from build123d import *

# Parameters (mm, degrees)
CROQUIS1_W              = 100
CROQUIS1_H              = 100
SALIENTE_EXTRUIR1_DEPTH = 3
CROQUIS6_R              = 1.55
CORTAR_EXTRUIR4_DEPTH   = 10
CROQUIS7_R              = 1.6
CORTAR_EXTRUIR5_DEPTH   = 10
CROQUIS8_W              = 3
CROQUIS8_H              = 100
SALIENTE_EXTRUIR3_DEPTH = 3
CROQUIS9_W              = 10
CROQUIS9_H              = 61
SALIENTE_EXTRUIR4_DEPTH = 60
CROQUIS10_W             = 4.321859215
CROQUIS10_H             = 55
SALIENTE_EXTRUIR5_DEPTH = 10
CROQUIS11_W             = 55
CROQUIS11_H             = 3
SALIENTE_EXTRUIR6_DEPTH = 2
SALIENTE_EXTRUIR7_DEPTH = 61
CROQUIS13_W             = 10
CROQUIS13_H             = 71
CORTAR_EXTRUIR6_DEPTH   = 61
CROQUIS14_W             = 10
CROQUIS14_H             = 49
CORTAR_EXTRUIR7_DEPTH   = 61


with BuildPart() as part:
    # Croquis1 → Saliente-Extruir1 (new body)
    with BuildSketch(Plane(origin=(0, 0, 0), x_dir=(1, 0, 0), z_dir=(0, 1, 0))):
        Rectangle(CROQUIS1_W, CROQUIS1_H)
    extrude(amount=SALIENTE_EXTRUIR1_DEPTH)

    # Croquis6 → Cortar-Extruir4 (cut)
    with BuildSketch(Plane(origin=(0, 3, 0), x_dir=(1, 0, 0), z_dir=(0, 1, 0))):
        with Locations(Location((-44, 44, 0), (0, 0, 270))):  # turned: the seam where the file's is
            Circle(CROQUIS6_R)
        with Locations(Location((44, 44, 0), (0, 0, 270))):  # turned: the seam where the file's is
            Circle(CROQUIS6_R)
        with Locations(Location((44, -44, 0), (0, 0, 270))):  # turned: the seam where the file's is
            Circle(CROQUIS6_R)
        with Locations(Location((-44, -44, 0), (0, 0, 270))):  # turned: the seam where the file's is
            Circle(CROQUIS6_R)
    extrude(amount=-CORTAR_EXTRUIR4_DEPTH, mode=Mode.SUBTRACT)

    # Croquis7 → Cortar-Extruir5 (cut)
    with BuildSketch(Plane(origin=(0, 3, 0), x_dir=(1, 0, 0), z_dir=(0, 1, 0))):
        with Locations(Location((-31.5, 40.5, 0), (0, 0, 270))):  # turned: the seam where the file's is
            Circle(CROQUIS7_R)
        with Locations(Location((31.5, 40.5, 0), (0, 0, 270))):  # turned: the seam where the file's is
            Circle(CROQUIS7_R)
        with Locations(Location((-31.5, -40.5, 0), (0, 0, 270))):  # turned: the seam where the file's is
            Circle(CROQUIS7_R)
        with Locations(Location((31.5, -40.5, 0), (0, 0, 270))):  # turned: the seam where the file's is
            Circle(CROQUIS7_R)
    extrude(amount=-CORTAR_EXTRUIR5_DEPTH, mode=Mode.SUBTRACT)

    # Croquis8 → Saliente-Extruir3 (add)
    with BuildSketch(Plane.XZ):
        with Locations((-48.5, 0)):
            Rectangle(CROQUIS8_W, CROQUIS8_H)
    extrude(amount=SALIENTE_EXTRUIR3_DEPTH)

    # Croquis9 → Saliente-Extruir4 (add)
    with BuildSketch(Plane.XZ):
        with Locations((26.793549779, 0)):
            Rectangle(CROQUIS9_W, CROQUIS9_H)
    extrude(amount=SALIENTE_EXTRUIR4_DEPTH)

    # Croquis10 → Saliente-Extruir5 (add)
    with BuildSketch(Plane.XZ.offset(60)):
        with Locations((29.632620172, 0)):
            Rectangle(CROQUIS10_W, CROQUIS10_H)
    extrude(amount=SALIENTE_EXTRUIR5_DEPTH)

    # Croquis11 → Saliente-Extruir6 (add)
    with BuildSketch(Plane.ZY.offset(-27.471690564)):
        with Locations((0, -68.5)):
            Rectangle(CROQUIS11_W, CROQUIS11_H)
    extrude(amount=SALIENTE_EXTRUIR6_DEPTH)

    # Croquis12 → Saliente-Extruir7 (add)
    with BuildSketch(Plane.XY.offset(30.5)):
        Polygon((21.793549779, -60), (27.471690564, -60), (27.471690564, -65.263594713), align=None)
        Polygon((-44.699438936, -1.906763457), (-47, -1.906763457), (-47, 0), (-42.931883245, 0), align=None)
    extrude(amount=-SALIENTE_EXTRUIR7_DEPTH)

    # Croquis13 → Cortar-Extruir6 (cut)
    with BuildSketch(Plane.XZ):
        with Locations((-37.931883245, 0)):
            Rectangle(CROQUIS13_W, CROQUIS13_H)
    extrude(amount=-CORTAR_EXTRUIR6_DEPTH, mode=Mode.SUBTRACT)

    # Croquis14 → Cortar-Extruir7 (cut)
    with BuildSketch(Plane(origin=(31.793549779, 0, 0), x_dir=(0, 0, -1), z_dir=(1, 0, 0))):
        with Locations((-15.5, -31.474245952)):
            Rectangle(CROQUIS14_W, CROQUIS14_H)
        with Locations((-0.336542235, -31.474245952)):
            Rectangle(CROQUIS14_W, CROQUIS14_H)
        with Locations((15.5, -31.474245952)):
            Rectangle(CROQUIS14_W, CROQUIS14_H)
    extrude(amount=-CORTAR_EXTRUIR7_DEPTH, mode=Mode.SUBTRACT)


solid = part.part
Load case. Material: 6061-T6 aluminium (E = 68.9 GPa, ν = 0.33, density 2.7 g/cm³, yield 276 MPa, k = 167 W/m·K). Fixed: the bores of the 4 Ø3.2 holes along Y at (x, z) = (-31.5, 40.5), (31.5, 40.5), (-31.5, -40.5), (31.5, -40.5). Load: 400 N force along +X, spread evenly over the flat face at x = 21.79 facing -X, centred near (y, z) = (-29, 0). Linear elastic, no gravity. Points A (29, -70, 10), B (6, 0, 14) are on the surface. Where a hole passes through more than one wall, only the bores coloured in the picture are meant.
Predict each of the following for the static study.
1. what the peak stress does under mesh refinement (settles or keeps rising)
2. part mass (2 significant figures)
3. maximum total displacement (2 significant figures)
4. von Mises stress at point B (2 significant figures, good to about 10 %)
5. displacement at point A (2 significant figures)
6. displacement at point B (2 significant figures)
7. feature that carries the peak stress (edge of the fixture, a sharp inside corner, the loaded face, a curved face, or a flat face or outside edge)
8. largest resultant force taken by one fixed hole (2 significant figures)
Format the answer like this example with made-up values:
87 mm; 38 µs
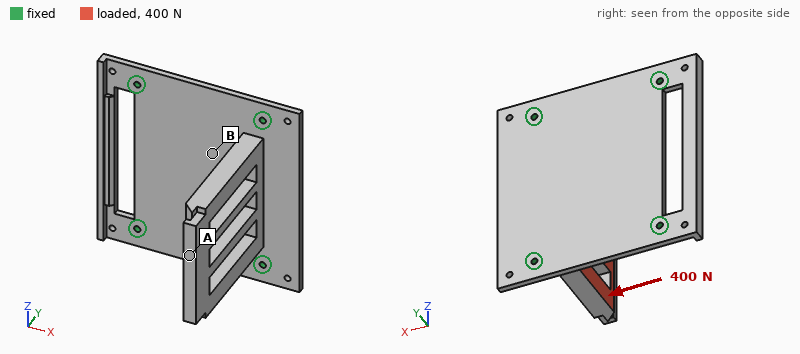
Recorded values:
keeps rising; 150 g; 0.48 mm; 24 MPa; 0.48 mm; 0.083 mm; edge of the fixture; 160 N
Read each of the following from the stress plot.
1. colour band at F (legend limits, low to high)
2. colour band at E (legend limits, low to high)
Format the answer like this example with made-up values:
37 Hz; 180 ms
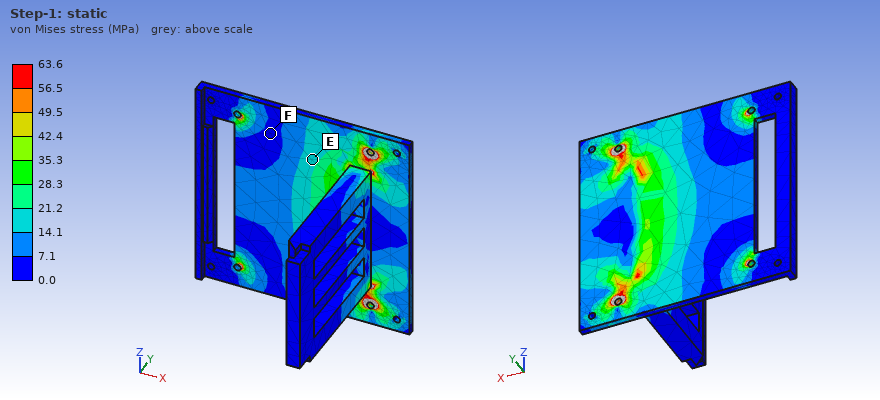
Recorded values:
0.0 to 7.1 MPa; 14.1 to 21.2 MPa
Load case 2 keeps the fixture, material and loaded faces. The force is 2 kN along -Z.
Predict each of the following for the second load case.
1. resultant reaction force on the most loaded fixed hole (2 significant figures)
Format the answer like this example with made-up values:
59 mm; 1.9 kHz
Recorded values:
1.2 kN
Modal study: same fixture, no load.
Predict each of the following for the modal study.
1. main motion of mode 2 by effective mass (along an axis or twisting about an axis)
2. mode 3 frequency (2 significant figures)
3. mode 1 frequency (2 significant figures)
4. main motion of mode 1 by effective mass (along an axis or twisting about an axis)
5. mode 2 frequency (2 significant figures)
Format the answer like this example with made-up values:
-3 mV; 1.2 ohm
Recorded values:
along Z; 2100 Hz; 610 Hz; along X; 1800 Hz
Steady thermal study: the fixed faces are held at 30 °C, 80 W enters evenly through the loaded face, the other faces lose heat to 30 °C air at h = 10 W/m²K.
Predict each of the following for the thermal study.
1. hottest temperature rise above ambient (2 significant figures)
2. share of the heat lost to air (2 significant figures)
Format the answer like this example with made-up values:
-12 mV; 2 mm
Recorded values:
76 K; 12 %
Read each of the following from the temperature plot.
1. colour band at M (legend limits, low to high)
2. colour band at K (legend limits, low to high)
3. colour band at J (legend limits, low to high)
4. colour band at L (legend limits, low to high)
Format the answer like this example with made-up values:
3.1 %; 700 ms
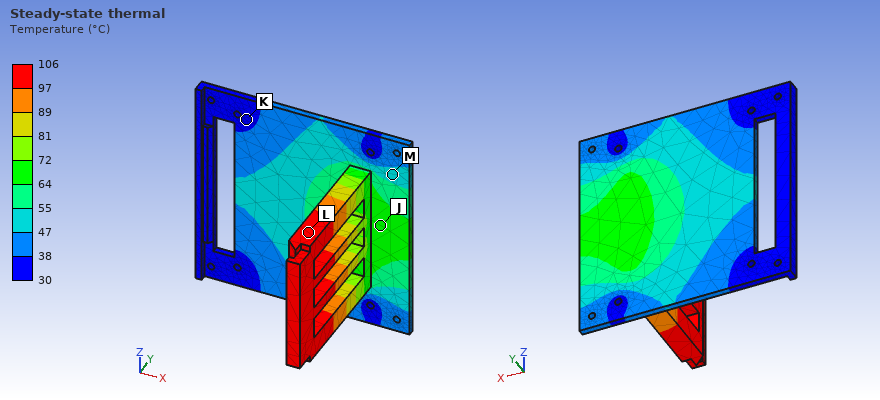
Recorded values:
47 to 55 °C; 30 to 38 °C; 64 to 72 °C; 97 to 106 °C
